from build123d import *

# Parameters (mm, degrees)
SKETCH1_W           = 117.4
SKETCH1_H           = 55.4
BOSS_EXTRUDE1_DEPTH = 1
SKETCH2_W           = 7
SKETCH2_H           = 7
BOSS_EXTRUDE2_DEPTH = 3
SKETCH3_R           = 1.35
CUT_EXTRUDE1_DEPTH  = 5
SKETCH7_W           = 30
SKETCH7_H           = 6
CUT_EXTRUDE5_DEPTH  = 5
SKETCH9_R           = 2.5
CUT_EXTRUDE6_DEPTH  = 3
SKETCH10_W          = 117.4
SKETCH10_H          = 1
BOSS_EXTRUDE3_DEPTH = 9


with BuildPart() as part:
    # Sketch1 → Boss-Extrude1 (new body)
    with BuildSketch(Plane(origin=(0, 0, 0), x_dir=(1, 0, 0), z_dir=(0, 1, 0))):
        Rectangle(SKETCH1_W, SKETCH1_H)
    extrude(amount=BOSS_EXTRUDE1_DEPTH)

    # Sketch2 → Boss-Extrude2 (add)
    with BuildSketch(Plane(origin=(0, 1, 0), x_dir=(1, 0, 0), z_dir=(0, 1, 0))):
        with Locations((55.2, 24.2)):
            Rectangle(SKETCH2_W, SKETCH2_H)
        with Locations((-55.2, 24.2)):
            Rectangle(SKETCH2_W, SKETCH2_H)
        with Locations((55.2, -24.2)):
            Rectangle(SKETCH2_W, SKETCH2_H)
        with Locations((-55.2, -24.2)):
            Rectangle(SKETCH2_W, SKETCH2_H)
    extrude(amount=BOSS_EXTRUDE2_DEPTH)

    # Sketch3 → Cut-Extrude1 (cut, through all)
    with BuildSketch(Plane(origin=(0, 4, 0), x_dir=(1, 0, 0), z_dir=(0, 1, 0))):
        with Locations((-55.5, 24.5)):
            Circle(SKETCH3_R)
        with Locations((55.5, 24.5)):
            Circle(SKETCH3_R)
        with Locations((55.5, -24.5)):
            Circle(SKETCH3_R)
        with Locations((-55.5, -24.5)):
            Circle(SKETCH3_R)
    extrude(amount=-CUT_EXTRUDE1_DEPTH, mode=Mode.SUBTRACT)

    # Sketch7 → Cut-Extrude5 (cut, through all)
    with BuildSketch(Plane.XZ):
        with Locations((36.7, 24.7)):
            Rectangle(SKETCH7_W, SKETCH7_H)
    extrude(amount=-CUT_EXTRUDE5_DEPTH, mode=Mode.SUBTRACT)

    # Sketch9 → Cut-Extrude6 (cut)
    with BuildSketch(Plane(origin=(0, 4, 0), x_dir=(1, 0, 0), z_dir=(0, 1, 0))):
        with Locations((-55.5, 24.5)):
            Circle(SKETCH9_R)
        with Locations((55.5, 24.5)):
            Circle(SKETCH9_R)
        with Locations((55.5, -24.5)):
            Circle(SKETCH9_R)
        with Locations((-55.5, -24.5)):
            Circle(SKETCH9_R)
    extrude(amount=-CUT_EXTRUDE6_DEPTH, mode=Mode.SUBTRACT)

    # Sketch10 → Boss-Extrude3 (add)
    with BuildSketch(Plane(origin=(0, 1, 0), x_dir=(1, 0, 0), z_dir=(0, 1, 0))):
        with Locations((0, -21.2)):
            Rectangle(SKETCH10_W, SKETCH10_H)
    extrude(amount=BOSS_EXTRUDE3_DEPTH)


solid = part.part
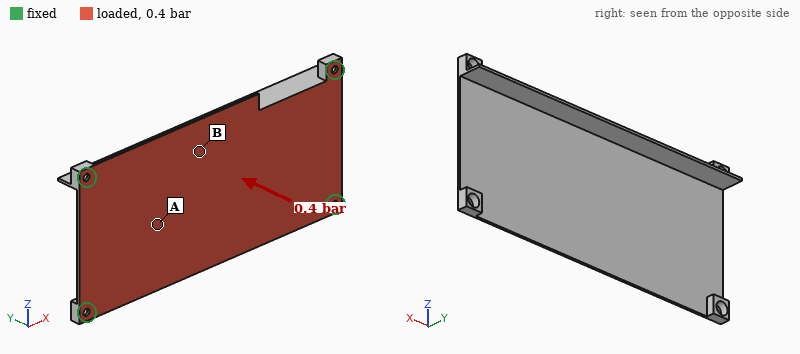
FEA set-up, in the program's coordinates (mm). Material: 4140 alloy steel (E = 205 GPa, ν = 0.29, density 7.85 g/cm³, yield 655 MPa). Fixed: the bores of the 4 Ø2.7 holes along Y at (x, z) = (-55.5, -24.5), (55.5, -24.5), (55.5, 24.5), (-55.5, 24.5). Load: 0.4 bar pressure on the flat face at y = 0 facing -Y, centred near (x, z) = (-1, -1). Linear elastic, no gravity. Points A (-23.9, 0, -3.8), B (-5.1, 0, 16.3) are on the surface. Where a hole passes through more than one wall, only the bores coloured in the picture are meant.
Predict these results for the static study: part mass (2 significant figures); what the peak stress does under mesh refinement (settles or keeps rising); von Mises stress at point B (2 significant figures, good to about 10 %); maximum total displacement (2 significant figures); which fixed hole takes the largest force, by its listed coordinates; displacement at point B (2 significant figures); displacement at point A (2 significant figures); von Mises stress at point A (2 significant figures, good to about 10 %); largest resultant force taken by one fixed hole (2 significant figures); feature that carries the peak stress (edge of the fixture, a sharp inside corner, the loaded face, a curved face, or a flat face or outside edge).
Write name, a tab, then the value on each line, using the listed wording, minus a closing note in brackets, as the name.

part mass	60 g
what the peak stress does under mesh refinement	keeps rising
von Mises stress at point B	24 MPa
maximum total displacement	0.75 mm
which fixed hole takes the largest force, by its listed coordinates	(-55.5, 24.5)
displacement at point B	0.12 mm
displacement at point A	0.32 mm
von Mises stress at point A	65 MPa
largest resultant force taken by one fixed hole	130 N
feature that carries the peak stress	edge of the fixture
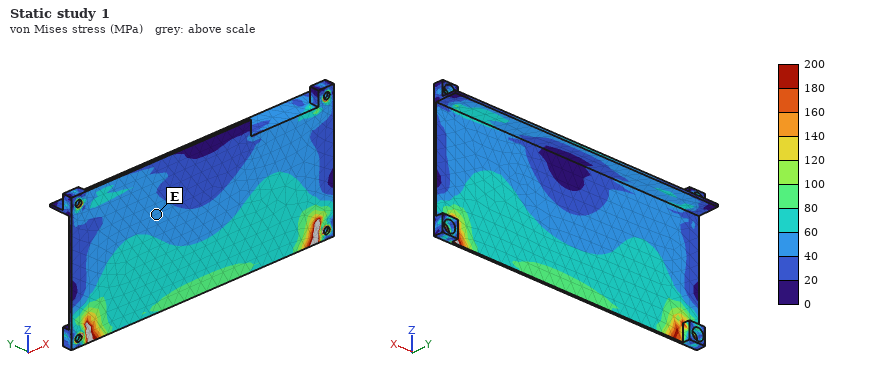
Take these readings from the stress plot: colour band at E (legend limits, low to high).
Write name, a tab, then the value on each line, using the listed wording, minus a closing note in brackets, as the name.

colour band at E	40 to 60 MPa
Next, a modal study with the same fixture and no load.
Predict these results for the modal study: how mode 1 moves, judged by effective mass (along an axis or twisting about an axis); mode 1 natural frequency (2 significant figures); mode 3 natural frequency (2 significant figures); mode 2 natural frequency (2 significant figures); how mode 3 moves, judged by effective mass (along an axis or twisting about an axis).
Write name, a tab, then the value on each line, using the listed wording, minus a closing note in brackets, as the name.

how mode 1 moves, judged by effective mass	along Y
mode 1 natural frequency	560 Hz
mode 3 natural frequency	1600 Hz
mode 2 natural frequency	1400 Hz
how mode 3 moves, judged by effective mass	along Y
